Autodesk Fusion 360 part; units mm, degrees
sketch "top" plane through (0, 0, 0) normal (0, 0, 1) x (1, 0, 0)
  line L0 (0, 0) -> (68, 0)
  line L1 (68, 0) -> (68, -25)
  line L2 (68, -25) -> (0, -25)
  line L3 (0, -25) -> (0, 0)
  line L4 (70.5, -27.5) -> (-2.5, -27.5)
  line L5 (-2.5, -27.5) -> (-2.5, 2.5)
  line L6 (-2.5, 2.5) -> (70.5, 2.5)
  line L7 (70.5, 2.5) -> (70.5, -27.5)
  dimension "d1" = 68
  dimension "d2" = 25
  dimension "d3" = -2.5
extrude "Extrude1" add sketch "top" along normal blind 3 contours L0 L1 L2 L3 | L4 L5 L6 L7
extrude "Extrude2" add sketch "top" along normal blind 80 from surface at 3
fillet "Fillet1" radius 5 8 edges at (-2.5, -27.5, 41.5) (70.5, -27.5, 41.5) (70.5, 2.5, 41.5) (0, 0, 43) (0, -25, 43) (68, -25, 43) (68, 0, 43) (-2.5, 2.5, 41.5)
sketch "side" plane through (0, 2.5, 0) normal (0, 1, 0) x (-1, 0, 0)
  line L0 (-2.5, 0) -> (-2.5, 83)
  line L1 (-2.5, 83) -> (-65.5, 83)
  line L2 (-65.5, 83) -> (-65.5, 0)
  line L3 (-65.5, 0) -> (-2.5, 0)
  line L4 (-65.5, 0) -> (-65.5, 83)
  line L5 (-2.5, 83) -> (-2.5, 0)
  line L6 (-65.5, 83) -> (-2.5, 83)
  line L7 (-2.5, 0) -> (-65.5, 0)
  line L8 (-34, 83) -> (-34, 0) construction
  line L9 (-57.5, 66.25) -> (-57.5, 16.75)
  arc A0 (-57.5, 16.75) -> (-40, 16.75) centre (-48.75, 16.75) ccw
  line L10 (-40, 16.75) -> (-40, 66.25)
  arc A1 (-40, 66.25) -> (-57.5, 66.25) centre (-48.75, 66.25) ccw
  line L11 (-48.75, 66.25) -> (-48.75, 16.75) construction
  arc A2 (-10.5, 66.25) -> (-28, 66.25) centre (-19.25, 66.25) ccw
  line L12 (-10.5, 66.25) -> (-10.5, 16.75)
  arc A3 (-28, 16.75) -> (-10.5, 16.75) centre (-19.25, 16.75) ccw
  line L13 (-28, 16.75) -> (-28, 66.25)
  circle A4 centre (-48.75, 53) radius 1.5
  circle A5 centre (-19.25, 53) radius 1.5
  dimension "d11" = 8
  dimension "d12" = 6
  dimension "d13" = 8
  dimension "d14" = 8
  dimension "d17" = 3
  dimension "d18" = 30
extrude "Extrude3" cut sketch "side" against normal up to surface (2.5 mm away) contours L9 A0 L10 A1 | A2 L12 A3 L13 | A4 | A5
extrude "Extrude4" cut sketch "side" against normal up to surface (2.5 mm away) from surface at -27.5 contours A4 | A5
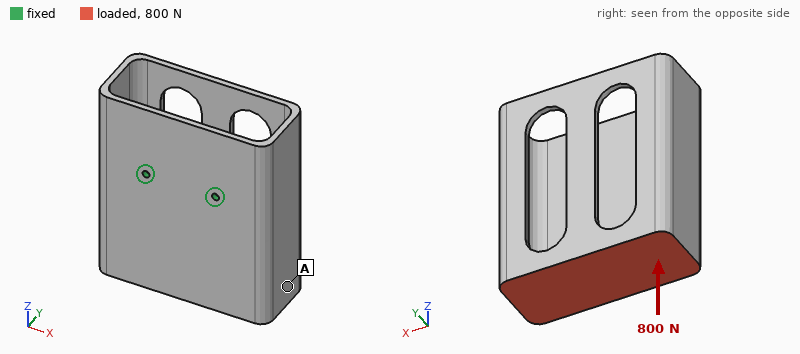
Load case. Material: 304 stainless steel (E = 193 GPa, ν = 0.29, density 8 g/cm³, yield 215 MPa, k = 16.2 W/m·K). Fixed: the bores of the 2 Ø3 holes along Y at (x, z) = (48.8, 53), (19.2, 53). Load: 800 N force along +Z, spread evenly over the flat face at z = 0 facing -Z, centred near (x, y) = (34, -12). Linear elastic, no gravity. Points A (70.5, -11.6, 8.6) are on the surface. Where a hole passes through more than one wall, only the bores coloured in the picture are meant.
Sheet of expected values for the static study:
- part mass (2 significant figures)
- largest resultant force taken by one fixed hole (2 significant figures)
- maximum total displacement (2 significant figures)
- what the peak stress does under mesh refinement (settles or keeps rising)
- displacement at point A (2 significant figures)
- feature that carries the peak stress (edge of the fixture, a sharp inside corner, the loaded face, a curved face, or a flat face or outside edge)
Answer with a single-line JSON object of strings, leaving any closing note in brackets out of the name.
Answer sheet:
{"part mass": "320 g", "largest resultant force taken by one fixed hole": "400 N", "maximum total displacement": "0.30 mm", "what the peak stress does under mesh refinement": "keeps rising", "displacement at point A": "0.23 mm", "feature that carries the peak stress": "edge of the fixture"}
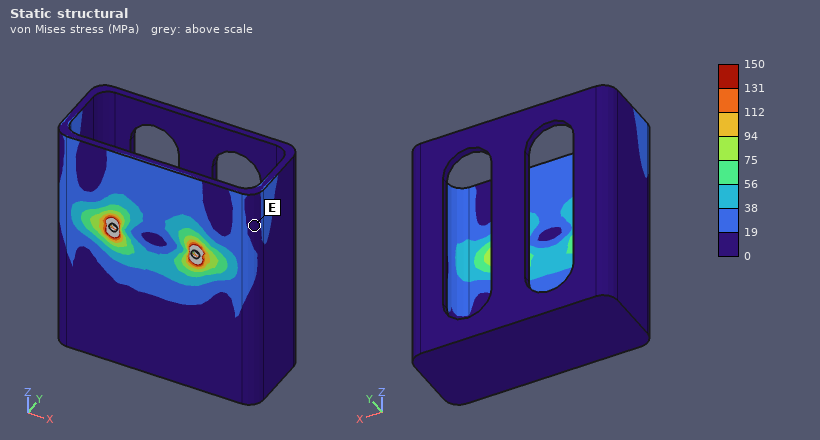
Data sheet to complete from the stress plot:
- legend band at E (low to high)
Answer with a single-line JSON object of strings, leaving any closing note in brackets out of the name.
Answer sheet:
{"legend band at E": "0 to 19 MPa"}
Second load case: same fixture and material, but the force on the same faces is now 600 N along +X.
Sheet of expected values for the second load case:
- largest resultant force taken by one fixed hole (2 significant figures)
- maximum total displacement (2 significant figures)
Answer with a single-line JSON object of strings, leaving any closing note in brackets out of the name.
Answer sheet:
{"largest resultant force taken by one fixed hole": "1.1 kN", "maximum total displacement": "85 µm"}
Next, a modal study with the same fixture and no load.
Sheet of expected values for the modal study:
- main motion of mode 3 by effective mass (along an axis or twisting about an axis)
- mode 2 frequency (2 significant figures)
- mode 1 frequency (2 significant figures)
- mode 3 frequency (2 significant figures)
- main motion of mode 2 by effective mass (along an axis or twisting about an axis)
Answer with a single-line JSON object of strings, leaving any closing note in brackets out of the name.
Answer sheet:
{"main motion of mode 3 by effective mass": "along Y", "mode 2 frequency": "690 Hz", "mode 1 frequency": "380 Hz", "mode 3 frequency": "1300 Hz", "main motion of mode 2 by effective mass": "along X"}
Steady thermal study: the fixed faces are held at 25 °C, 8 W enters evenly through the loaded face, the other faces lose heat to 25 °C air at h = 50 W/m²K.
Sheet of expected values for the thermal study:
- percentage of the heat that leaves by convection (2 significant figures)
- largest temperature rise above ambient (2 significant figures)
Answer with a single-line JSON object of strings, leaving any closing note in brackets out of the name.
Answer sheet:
{"percentage of the heat that leaves by convection": "97 %", "largest temperature rise above ambient": "24 K"}
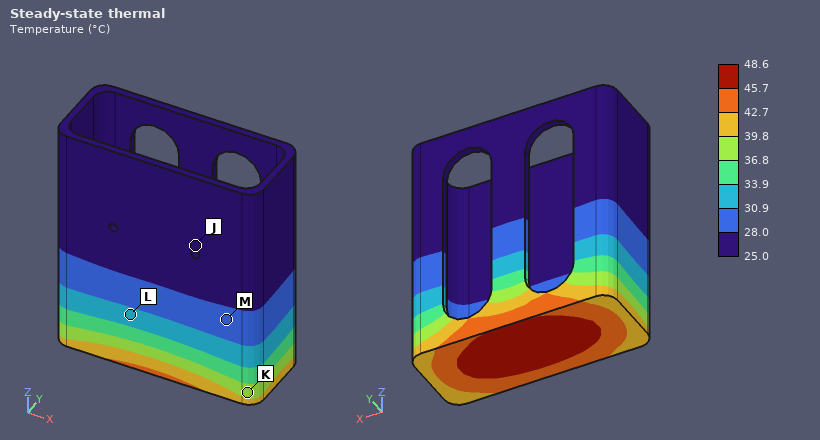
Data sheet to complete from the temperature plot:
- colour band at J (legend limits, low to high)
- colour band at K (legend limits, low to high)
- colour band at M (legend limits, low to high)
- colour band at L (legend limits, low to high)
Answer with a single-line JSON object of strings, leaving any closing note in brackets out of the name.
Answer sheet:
{"colour band at J": "25.0 to 28.0 °C", "colour band at K": "36.8 to 39.8 °C", "colour band at M": "28.0 to 30.9 °C", "colour band at L": "30.9 to 33.9 °C"}
